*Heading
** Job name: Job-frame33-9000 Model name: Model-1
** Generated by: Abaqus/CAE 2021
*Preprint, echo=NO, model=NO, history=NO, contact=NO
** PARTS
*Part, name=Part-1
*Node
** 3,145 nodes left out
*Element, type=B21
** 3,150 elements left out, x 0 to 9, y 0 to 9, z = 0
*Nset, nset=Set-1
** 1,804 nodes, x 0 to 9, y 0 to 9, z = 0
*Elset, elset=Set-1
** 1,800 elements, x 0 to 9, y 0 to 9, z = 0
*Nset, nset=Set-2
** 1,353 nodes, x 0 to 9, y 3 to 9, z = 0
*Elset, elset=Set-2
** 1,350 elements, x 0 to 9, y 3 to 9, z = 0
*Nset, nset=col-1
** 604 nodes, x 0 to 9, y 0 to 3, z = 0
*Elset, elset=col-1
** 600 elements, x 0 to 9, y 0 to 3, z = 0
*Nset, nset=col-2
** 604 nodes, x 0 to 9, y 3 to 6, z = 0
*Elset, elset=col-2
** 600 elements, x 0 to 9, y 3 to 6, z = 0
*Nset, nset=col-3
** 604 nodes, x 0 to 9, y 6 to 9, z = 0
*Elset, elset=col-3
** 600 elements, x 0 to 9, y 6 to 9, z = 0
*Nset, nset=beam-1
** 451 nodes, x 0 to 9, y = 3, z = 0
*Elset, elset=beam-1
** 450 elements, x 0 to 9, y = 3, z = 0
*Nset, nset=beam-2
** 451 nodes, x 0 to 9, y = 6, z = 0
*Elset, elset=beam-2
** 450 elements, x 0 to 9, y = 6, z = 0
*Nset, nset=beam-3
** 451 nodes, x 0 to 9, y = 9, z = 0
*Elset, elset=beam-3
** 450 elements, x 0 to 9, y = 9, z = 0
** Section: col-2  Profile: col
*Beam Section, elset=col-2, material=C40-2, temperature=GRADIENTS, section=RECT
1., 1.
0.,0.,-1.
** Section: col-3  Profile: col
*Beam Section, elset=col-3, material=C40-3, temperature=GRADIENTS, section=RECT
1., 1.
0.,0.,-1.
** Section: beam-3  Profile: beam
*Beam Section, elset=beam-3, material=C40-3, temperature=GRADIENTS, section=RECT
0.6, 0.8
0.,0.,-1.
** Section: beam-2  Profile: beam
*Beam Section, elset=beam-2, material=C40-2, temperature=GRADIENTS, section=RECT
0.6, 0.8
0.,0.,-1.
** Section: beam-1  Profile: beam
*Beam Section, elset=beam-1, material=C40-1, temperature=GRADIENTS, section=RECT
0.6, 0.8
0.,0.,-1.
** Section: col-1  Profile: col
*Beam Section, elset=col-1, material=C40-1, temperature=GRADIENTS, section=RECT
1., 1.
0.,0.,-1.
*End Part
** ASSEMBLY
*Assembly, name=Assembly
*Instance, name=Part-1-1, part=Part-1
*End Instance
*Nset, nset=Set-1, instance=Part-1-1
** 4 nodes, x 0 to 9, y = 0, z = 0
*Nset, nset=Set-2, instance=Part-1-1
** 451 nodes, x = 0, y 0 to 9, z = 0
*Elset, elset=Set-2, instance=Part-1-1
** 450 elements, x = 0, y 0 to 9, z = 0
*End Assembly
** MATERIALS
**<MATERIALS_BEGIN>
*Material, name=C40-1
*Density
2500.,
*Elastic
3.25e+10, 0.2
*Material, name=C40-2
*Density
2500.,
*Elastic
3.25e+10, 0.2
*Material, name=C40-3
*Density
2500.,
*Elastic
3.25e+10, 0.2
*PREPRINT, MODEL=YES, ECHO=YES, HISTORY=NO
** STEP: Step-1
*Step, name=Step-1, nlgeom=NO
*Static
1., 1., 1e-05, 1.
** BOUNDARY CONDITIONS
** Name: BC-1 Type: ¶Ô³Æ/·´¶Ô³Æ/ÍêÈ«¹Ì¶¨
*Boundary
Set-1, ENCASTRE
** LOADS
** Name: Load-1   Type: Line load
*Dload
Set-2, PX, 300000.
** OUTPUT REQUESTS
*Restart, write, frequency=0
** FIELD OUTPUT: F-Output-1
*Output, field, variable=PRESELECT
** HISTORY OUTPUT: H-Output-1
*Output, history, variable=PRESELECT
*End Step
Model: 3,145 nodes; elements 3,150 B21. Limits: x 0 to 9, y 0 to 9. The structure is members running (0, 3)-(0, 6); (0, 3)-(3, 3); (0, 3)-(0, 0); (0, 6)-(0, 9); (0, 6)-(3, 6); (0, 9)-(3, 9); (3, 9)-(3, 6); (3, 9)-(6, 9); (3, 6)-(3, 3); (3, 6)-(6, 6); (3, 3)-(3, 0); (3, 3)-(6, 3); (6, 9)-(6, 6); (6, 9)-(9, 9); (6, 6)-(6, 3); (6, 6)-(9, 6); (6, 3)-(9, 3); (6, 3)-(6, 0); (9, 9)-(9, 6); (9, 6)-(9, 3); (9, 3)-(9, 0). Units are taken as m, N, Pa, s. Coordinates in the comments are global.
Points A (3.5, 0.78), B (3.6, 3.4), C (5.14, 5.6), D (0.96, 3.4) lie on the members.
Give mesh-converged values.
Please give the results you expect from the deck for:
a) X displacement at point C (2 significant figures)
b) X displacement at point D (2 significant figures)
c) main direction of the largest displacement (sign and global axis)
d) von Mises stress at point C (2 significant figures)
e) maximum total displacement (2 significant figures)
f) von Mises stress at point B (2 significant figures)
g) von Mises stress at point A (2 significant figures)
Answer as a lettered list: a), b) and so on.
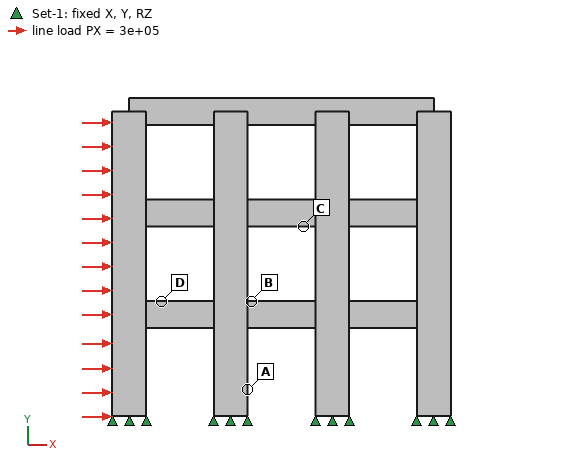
a) 0.0027 m
b) 0.0013 m
c) +X
d) 3.9e+06 Pa
e) 0.0036 m
f) 6.2e+06 Pa
g) 4.9e+06 Pa
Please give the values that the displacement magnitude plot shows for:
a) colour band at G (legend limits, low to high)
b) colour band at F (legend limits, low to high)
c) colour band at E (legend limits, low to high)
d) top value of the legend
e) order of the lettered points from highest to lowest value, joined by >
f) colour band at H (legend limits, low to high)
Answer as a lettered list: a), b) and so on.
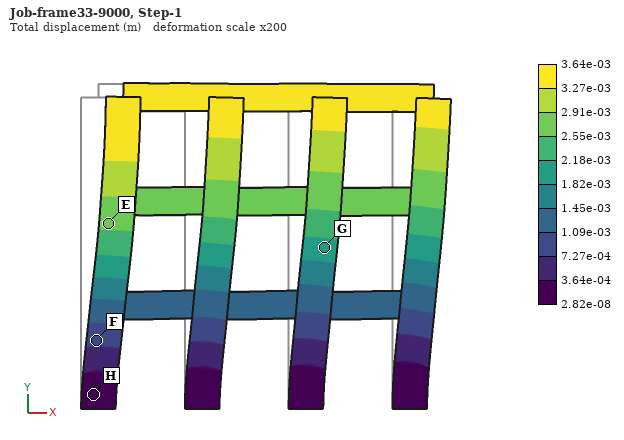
a) 1.82e-03 to 2.18e-03 m
b) 7.27e-04 to 1.09e-03 m
c) 2.55e-03 to 2.91e-03 m
d) 3.64e-03 m
e) E > G > F > H
f) 2.82e-08 to 3.64e-04 m
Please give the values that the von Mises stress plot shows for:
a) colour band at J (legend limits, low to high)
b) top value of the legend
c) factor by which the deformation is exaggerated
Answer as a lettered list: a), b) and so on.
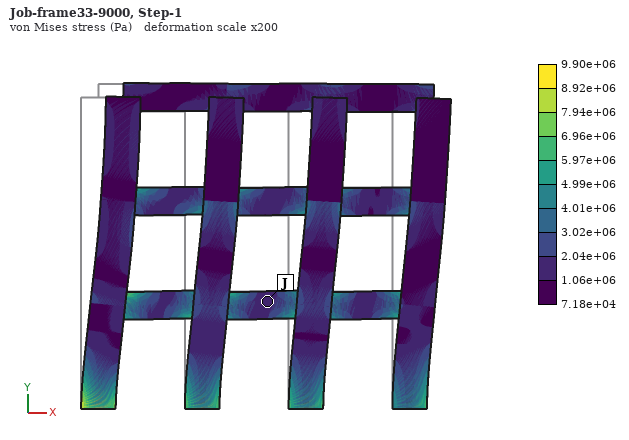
a) 1.06e+06 to 2.04e+06 Pa
b) 9.90e+06 Pa
c) 200
